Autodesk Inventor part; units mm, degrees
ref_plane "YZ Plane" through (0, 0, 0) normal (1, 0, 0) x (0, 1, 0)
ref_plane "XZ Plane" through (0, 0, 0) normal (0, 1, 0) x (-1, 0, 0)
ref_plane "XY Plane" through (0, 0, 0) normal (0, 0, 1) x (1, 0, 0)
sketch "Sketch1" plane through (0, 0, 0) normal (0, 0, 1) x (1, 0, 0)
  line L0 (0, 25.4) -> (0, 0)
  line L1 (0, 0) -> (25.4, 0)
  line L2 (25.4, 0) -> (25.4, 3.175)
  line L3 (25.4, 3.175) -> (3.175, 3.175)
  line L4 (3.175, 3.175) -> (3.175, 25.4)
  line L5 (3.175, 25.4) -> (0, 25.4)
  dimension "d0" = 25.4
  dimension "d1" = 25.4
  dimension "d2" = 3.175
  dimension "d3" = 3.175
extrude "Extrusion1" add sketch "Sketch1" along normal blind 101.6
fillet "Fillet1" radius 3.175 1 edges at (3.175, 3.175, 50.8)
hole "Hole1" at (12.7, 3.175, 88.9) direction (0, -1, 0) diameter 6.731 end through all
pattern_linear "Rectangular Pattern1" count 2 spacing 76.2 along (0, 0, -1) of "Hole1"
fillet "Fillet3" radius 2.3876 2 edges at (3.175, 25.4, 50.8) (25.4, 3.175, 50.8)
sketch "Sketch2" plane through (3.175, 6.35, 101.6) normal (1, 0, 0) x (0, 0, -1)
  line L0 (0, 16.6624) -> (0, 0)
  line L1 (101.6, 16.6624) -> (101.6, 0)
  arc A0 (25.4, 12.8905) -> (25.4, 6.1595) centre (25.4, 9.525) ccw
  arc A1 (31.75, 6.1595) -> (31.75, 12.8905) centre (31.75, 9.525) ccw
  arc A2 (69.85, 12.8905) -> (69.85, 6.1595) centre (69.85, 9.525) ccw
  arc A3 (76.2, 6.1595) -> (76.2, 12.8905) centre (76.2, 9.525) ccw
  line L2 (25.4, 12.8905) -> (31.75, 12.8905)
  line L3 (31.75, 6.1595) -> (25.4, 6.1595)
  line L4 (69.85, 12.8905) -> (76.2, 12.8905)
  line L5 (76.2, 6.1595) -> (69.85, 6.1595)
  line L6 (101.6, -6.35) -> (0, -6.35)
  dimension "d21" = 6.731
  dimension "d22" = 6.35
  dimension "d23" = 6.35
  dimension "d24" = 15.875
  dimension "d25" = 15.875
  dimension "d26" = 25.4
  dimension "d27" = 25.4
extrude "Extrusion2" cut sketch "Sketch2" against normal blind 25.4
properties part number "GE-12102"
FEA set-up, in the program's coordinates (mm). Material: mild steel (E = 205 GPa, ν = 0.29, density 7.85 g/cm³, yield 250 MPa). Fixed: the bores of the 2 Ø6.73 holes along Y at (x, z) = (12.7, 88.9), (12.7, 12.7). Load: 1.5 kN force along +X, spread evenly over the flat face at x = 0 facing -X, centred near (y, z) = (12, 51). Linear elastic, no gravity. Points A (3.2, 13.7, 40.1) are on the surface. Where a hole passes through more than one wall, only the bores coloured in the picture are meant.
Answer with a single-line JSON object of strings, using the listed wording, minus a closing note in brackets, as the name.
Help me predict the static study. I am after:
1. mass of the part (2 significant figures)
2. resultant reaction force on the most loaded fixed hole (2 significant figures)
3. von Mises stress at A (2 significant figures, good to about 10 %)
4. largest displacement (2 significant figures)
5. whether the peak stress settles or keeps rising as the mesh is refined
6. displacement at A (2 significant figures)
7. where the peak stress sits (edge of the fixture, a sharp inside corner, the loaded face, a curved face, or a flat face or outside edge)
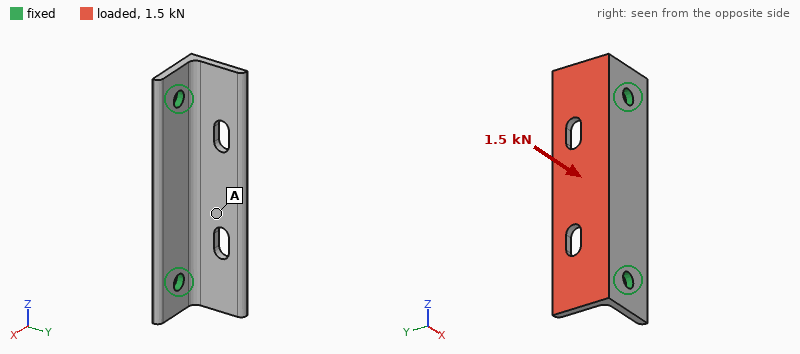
{"mass of the part": "110 g", "resultant reaction force on the most loaded fixed hole": "750 N", "von Mises stress at A": "32 MPa", "largest displacement": "0.13 mm", "whether the peak stress settles or keeps rising as the mesh is refined": "keeps rising", "displacement at A": "0.062 mm", "where the peak stress sits": "edge of the fixture"}
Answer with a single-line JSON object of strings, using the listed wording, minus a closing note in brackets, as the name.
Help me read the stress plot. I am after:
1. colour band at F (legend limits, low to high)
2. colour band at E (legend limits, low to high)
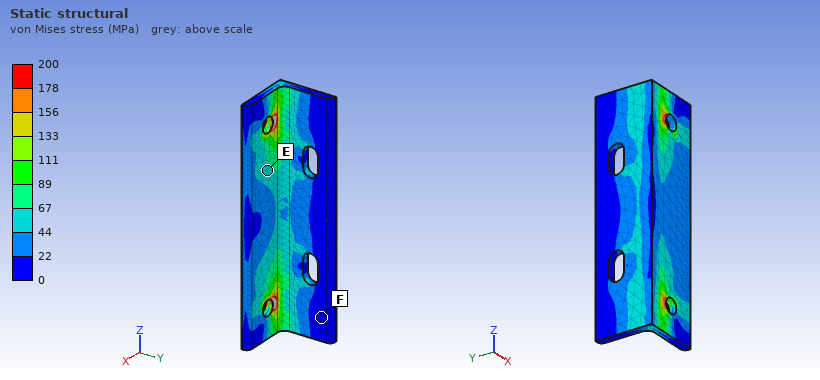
{"colour band at F": "0 to 22 MPa", "colour band at E": "44 to 67 MPa"}
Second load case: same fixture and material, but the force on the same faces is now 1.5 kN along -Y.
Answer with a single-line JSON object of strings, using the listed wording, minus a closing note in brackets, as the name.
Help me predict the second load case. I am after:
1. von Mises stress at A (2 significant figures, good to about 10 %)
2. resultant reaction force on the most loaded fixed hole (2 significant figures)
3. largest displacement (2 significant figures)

{"von Mises stress at A": "17 MPa", "resultant reaction force on the most loaded fixed hole": "790 N", "largest displacement": "70 µm"}
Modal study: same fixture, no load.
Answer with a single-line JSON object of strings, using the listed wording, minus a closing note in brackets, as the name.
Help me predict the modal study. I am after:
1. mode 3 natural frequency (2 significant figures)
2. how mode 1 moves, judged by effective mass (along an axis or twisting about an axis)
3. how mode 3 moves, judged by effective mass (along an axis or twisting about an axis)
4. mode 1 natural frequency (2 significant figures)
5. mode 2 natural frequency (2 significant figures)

{"mode 3 natural frequency": "4700 Hz", "how mode 1 moves, judged by effective mass": "along X", "how mode 3 moves, judged by effective mass": "along Y", "mode 1 natural frequency": "2600 Hz", "mode 2 natural frequency": "3900 Hz"}
